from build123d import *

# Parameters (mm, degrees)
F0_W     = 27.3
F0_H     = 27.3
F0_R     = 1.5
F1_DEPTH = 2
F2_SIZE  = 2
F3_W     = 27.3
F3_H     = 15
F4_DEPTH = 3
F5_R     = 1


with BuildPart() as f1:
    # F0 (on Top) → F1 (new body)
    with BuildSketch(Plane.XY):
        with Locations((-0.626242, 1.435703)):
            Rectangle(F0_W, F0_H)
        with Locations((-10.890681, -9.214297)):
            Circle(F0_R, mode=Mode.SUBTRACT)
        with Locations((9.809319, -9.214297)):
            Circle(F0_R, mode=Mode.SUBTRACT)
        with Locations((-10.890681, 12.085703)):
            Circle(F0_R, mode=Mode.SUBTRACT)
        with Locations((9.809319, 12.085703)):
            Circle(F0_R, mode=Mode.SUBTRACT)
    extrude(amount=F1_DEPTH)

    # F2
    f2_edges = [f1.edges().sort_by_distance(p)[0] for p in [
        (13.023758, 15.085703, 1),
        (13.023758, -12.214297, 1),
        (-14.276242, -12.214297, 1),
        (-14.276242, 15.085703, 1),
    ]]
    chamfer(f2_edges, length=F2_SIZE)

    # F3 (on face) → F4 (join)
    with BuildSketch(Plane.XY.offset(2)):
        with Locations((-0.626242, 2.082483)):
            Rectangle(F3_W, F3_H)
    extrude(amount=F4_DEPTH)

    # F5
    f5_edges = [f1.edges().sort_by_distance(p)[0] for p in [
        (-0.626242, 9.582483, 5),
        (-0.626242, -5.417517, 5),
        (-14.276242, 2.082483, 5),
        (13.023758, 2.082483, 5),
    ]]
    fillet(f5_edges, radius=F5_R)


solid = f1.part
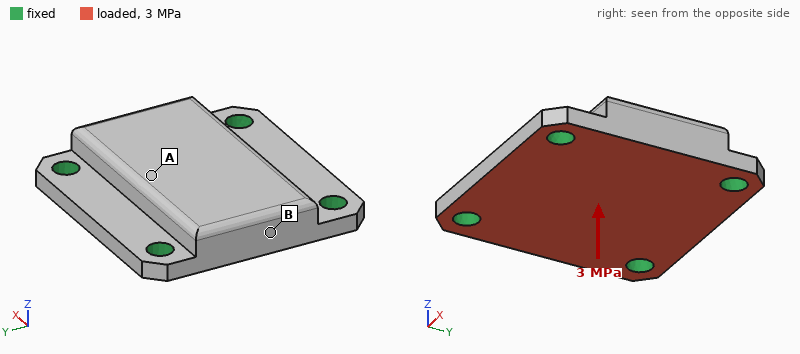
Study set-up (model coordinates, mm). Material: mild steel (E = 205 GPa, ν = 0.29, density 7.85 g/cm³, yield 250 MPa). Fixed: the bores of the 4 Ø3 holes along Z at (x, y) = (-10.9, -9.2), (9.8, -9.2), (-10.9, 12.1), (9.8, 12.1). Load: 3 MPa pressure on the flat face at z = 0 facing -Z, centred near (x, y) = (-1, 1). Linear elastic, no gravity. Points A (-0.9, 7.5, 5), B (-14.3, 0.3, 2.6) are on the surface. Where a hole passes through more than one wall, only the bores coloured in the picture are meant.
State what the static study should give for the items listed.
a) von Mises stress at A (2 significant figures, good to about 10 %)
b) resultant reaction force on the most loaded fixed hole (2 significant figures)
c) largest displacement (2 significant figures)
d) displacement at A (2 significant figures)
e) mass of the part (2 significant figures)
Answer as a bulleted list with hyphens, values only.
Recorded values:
- 37 MPa
- 580 N
- 7.1 µm
- 4.8 µm
- 21 g
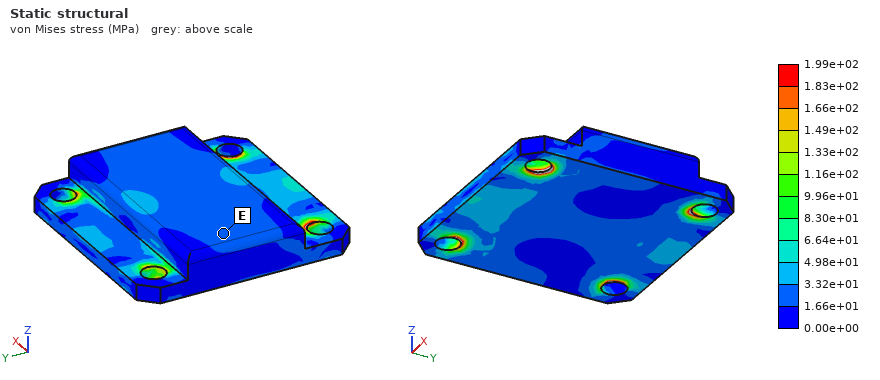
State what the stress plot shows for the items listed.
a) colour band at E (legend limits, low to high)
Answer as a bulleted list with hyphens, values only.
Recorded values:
- 1.66e+01 to 3.32e+01 MPa
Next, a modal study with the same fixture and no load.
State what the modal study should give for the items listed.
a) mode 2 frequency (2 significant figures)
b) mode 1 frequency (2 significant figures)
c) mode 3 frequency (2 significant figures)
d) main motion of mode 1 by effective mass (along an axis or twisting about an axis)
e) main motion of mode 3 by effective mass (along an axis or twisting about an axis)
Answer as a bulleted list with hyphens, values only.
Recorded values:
- 34 kHz
- 23 kHz
- 36 kHz
- along Z
- twisting about X
